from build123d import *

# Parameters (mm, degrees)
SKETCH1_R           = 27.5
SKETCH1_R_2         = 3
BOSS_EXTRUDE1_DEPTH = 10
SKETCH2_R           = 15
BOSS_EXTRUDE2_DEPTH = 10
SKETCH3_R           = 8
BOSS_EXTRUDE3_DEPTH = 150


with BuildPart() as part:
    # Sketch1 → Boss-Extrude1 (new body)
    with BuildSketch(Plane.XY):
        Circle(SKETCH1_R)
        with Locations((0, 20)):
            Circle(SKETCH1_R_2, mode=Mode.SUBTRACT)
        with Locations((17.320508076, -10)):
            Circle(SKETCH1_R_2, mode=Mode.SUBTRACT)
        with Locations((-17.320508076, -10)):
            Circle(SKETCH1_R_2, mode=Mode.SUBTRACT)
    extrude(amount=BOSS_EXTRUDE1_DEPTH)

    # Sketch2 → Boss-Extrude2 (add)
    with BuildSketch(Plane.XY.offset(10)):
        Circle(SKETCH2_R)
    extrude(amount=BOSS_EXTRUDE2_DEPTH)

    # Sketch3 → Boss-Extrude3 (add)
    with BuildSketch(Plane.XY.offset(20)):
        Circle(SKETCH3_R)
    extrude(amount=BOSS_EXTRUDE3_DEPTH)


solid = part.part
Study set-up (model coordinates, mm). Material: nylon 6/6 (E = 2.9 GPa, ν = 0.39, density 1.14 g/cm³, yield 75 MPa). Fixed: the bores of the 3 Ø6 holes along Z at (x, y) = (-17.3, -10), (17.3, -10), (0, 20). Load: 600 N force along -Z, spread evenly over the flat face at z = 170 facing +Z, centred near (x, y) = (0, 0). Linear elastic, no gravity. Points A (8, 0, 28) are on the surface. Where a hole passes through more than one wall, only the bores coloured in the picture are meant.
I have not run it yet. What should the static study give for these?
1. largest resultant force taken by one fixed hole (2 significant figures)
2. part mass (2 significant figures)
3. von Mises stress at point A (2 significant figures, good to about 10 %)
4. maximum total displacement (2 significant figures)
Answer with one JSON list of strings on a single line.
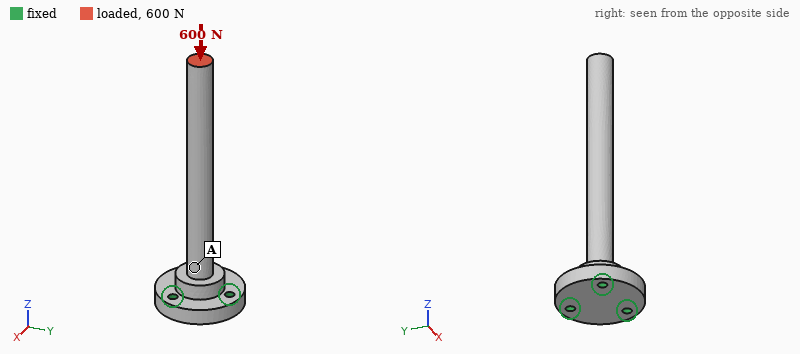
["210 N", "69 g", "2.9 MPa", "0.17 mm"]
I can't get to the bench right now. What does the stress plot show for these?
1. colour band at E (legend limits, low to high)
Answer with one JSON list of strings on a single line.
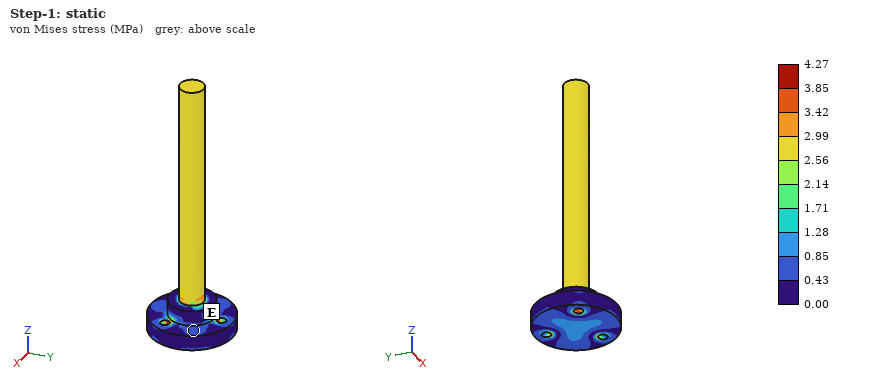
["0.43 to 0.85 MPa"]
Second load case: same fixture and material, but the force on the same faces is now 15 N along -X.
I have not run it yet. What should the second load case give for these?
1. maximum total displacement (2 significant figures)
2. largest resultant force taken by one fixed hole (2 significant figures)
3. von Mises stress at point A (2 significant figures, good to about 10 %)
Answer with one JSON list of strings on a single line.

["2.0 mm", "69 N", "5.2 MPa"]
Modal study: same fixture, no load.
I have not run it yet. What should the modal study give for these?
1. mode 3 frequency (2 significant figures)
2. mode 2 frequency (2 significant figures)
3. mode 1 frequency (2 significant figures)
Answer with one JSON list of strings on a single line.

["900 Hz", "150 Hz", "150 Hz"]
